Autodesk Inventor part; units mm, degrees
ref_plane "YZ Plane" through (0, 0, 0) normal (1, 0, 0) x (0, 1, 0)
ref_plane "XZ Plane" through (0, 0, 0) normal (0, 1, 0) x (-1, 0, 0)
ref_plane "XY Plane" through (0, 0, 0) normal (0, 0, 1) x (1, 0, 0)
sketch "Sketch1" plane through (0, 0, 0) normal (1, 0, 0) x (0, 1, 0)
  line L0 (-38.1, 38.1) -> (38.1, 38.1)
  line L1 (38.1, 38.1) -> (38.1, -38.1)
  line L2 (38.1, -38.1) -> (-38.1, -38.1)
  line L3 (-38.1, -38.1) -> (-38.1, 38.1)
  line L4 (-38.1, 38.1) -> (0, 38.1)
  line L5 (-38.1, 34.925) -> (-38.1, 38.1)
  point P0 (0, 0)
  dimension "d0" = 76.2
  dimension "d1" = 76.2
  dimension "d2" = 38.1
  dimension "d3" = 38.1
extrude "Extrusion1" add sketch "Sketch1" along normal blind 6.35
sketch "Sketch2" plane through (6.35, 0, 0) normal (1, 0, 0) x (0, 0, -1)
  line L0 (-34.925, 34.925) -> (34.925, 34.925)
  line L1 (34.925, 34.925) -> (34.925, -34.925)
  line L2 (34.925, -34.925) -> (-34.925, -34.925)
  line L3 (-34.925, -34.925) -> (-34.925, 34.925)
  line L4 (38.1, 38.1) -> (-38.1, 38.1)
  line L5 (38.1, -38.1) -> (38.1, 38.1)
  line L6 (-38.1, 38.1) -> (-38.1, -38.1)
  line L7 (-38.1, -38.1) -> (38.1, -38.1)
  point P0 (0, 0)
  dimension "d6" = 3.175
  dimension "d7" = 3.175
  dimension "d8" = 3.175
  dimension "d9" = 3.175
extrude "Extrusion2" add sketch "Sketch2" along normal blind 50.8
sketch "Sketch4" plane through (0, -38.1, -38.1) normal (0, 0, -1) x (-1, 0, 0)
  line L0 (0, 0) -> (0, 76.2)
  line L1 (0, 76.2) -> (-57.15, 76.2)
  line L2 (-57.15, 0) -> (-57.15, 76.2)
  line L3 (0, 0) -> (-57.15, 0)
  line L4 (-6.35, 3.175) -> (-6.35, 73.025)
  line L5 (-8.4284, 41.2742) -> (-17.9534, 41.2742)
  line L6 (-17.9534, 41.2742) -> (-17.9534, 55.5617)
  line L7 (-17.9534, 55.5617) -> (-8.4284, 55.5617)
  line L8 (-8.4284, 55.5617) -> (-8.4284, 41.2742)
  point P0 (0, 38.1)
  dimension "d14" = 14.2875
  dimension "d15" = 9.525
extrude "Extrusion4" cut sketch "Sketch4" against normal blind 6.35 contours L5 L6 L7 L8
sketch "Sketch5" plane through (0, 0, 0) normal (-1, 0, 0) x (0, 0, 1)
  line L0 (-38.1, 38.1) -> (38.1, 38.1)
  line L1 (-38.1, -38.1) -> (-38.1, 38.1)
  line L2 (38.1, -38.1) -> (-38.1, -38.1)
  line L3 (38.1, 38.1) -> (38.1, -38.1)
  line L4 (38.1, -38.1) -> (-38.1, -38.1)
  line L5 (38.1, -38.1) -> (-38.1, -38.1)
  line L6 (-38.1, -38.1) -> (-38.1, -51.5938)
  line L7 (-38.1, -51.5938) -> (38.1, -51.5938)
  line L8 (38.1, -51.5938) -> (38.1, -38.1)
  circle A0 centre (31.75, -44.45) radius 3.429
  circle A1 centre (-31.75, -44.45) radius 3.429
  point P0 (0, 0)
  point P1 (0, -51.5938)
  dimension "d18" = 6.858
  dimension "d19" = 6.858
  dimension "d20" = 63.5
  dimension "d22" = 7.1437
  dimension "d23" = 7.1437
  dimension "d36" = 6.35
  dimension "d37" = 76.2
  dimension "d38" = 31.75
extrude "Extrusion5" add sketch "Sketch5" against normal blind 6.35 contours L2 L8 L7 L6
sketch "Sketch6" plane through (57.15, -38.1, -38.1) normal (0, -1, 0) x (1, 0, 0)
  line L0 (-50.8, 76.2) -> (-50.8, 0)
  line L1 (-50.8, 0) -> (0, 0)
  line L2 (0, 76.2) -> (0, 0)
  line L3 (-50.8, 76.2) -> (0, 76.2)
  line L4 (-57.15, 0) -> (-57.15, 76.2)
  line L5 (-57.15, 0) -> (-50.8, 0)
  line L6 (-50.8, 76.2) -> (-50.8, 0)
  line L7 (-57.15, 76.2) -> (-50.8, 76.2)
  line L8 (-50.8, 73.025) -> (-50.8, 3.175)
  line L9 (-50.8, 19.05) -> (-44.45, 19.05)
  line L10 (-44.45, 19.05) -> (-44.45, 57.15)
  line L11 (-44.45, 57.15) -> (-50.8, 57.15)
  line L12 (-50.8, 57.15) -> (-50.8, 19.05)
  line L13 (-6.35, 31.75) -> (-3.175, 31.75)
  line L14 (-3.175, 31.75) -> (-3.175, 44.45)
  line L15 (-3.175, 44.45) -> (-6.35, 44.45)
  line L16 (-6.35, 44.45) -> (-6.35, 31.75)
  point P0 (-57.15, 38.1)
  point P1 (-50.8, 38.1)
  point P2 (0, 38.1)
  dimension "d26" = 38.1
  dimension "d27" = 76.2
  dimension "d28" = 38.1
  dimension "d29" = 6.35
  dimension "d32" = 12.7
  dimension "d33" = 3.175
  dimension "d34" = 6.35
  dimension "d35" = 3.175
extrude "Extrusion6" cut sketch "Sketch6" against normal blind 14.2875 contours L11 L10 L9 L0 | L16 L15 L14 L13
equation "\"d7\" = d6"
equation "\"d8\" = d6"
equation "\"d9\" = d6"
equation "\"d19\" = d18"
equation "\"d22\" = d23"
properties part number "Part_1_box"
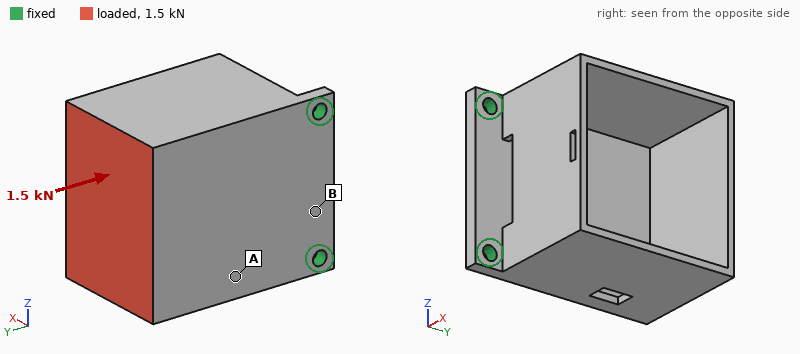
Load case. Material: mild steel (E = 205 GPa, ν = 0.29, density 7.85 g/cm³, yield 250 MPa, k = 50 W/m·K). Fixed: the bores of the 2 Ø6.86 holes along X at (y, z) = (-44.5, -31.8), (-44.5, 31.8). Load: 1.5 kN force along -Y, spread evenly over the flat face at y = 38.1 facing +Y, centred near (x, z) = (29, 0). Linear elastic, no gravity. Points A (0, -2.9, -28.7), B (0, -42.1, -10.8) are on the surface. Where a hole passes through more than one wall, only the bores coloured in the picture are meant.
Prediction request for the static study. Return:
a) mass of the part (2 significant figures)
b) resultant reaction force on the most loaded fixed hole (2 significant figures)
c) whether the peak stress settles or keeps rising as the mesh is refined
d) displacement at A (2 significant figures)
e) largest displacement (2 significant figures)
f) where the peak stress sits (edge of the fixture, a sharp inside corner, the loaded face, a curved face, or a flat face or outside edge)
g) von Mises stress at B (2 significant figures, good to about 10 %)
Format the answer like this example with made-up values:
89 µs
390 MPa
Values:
700 g
760 N
keeps rising
0.070 mm
0.25 mm
edge of the fixture
24 MPa
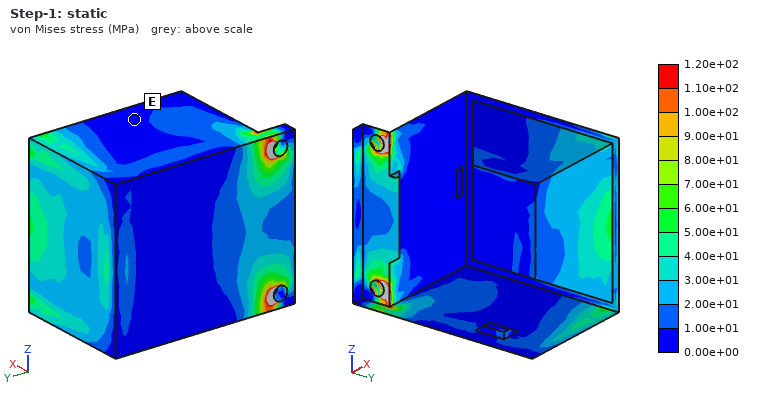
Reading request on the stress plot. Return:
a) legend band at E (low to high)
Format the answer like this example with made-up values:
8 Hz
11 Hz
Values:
0.00e+00 to 1.00e+01 MPa
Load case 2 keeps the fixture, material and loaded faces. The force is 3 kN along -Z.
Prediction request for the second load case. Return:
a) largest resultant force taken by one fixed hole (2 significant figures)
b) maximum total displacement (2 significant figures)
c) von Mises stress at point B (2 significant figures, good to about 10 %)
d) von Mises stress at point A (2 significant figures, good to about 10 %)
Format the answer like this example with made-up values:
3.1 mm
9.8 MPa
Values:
4.3 kN
0.35 mm
22 MPa
49 MPa
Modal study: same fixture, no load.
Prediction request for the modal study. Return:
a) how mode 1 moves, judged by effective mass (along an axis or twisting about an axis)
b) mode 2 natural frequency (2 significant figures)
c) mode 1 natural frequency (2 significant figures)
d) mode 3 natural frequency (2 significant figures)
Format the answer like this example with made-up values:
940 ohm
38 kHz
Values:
along X
980 Hz
510 Hz
2200 Hz
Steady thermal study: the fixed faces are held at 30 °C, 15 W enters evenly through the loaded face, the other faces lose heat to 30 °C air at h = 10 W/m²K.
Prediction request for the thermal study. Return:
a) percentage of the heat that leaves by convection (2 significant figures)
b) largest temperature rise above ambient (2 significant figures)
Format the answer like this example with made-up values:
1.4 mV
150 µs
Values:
42 %
38 K
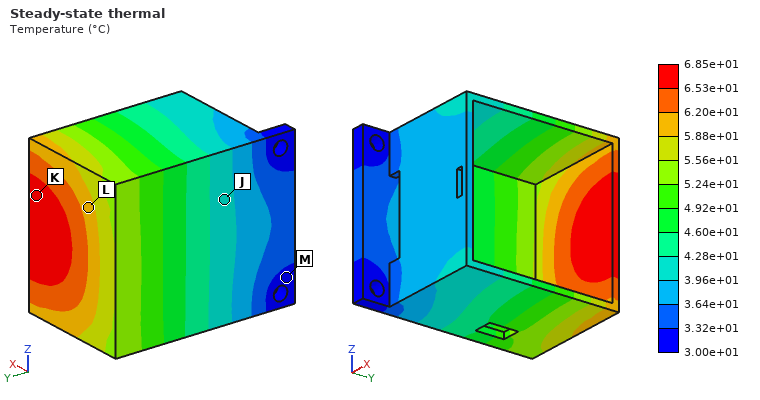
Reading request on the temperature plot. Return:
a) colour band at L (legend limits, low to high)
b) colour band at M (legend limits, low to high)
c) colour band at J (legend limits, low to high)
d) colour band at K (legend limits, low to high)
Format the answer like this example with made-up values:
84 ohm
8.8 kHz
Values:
5.88e+01 to 6.20e+01 °C
3.00e+01 to 3.32e+01 °C
3.96e+01 to 4.28e+01 °C
6.53e+01 to 6.85e+01 °C
